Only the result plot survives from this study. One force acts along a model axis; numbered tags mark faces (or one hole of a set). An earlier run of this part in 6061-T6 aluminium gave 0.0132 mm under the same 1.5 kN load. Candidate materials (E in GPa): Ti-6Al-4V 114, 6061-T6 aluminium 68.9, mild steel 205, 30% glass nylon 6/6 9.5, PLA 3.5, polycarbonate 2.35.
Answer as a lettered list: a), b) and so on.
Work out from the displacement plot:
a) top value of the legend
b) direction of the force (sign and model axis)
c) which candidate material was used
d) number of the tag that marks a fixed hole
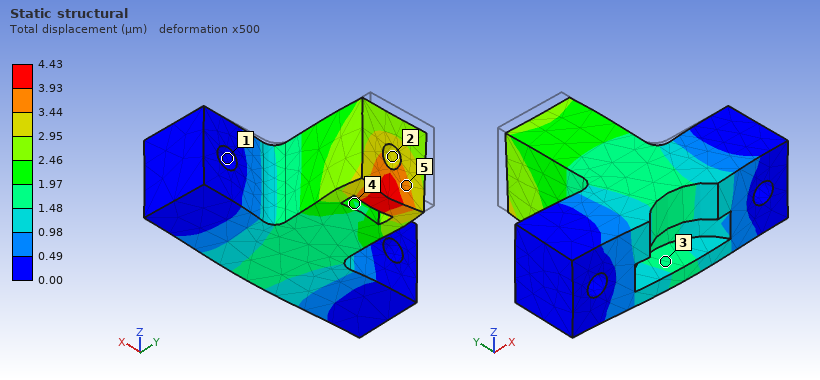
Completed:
a) 4.43 µm
b) -Y
c) mild steel
d) 1
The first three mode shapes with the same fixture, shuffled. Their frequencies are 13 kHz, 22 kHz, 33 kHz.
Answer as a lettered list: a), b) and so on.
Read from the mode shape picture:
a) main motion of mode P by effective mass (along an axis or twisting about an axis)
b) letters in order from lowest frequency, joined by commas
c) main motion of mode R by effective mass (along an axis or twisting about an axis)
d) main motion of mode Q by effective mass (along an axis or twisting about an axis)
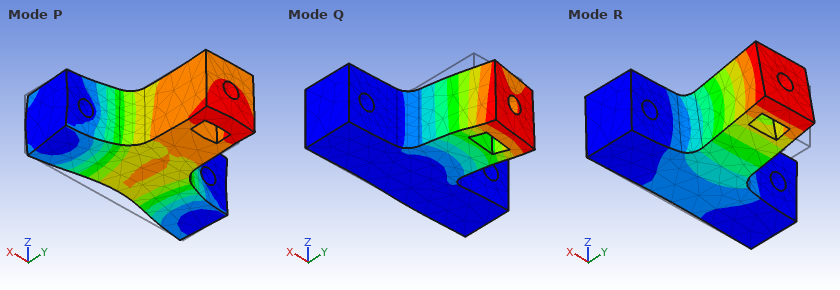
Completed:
a) along Y
b) R, Q, P
c) along Z
d) along X
